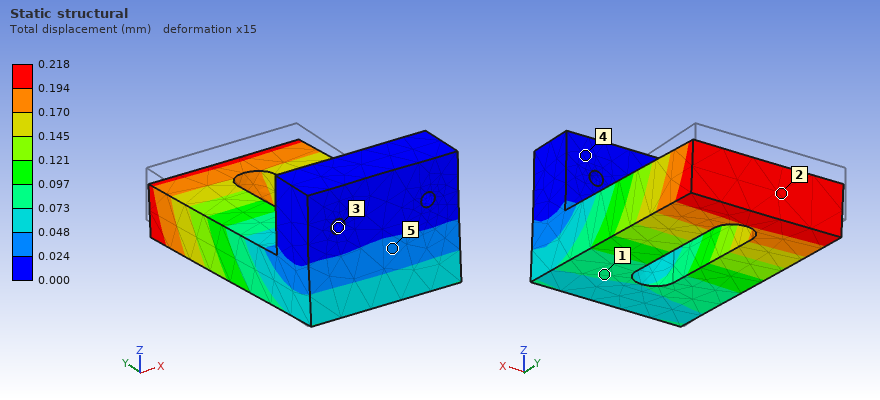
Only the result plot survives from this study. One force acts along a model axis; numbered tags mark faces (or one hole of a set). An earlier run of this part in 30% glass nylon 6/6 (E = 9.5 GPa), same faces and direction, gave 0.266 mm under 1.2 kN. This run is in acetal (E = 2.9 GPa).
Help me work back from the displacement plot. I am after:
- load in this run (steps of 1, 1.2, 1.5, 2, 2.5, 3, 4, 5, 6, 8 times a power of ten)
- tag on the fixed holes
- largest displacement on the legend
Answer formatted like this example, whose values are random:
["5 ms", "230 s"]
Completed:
["300 N", "3", "0.218 mm"]
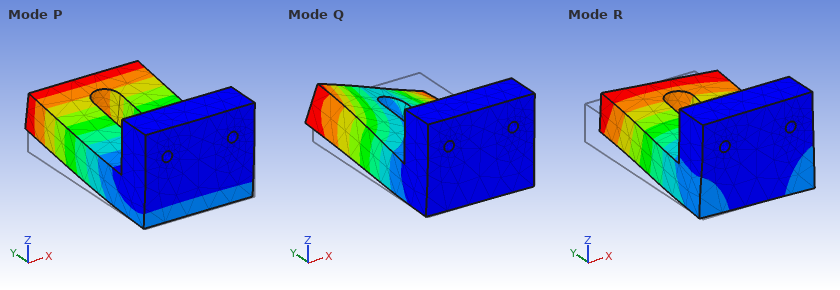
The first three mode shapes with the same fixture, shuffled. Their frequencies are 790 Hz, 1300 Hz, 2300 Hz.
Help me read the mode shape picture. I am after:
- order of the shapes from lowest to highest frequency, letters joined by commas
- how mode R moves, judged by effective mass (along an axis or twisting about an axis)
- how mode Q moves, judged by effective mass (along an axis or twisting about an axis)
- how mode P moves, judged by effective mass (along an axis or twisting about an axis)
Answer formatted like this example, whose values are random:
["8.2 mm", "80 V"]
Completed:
["P, R, Q", "along X", "twisting about Y", "along Z"]
